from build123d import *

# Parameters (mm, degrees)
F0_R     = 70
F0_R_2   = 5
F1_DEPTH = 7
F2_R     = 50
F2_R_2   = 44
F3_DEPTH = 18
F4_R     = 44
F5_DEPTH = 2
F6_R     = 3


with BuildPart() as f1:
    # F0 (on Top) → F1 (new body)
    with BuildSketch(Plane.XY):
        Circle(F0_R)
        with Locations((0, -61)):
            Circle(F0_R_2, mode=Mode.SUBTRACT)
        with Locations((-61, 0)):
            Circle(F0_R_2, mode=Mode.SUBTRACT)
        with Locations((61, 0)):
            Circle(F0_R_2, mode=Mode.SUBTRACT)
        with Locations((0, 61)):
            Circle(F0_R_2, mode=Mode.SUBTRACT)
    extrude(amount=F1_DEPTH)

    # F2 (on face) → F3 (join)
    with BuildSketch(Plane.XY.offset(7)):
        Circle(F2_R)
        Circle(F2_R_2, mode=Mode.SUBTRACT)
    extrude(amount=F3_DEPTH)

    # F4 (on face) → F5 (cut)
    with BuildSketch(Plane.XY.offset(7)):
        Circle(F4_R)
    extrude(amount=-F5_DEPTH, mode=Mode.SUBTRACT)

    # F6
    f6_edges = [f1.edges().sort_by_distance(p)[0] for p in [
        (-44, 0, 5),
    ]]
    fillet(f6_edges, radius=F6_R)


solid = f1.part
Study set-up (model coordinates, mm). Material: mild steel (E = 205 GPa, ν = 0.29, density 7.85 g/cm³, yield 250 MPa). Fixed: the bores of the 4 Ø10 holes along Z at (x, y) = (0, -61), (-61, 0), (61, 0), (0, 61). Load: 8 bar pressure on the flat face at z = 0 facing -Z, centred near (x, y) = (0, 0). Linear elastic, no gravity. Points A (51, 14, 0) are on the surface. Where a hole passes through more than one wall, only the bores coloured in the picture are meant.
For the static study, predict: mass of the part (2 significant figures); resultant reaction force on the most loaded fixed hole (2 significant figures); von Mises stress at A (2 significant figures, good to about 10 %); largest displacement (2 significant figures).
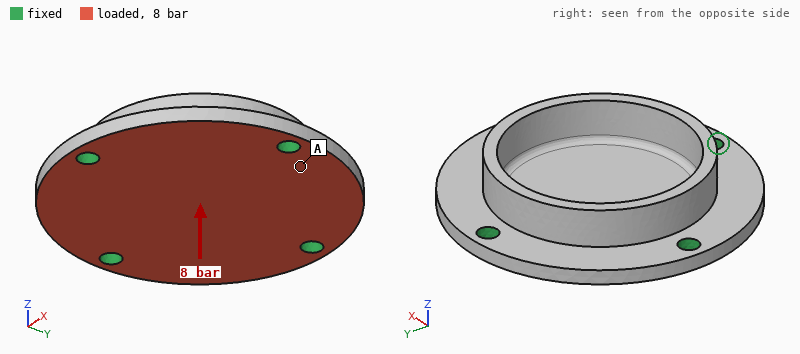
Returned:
990 g
3.0 kN
17 MPa
36 µm
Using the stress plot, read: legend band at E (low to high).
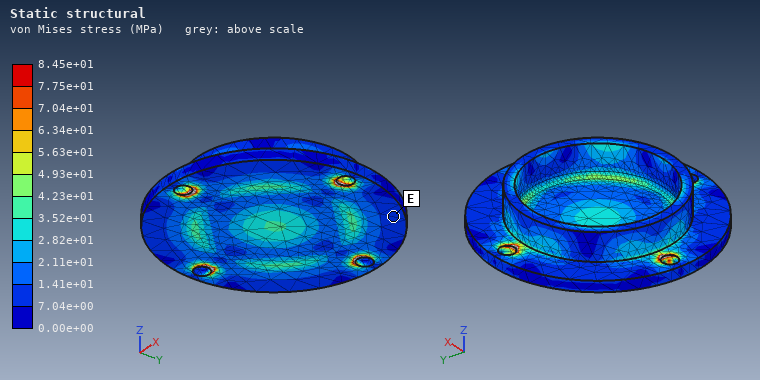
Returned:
7.04e+00 to 1.41e+01 MPa
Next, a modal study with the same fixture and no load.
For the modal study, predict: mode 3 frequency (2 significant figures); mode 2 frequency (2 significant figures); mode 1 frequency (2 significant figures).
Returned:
5500 Hz
4700 Hz
4600 Hz
